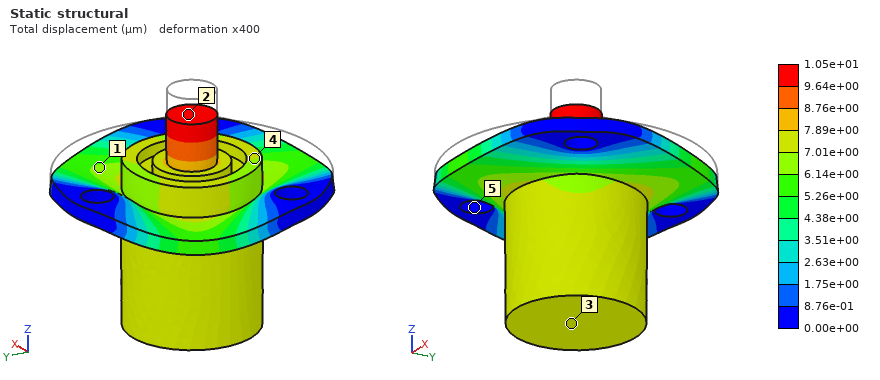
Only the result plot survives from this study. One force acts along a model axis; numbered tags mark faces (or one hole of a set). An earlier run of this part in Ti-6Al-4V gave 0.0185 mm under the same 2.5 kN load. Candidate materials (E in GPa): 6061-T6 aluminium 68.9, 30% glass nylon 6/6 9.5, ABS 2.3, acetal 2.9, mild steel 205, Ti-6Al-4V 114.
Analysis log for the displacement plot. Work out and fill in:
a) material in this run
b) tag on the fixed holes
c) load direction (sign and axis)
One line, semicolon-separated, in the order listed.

mild steel; 5; -Z
